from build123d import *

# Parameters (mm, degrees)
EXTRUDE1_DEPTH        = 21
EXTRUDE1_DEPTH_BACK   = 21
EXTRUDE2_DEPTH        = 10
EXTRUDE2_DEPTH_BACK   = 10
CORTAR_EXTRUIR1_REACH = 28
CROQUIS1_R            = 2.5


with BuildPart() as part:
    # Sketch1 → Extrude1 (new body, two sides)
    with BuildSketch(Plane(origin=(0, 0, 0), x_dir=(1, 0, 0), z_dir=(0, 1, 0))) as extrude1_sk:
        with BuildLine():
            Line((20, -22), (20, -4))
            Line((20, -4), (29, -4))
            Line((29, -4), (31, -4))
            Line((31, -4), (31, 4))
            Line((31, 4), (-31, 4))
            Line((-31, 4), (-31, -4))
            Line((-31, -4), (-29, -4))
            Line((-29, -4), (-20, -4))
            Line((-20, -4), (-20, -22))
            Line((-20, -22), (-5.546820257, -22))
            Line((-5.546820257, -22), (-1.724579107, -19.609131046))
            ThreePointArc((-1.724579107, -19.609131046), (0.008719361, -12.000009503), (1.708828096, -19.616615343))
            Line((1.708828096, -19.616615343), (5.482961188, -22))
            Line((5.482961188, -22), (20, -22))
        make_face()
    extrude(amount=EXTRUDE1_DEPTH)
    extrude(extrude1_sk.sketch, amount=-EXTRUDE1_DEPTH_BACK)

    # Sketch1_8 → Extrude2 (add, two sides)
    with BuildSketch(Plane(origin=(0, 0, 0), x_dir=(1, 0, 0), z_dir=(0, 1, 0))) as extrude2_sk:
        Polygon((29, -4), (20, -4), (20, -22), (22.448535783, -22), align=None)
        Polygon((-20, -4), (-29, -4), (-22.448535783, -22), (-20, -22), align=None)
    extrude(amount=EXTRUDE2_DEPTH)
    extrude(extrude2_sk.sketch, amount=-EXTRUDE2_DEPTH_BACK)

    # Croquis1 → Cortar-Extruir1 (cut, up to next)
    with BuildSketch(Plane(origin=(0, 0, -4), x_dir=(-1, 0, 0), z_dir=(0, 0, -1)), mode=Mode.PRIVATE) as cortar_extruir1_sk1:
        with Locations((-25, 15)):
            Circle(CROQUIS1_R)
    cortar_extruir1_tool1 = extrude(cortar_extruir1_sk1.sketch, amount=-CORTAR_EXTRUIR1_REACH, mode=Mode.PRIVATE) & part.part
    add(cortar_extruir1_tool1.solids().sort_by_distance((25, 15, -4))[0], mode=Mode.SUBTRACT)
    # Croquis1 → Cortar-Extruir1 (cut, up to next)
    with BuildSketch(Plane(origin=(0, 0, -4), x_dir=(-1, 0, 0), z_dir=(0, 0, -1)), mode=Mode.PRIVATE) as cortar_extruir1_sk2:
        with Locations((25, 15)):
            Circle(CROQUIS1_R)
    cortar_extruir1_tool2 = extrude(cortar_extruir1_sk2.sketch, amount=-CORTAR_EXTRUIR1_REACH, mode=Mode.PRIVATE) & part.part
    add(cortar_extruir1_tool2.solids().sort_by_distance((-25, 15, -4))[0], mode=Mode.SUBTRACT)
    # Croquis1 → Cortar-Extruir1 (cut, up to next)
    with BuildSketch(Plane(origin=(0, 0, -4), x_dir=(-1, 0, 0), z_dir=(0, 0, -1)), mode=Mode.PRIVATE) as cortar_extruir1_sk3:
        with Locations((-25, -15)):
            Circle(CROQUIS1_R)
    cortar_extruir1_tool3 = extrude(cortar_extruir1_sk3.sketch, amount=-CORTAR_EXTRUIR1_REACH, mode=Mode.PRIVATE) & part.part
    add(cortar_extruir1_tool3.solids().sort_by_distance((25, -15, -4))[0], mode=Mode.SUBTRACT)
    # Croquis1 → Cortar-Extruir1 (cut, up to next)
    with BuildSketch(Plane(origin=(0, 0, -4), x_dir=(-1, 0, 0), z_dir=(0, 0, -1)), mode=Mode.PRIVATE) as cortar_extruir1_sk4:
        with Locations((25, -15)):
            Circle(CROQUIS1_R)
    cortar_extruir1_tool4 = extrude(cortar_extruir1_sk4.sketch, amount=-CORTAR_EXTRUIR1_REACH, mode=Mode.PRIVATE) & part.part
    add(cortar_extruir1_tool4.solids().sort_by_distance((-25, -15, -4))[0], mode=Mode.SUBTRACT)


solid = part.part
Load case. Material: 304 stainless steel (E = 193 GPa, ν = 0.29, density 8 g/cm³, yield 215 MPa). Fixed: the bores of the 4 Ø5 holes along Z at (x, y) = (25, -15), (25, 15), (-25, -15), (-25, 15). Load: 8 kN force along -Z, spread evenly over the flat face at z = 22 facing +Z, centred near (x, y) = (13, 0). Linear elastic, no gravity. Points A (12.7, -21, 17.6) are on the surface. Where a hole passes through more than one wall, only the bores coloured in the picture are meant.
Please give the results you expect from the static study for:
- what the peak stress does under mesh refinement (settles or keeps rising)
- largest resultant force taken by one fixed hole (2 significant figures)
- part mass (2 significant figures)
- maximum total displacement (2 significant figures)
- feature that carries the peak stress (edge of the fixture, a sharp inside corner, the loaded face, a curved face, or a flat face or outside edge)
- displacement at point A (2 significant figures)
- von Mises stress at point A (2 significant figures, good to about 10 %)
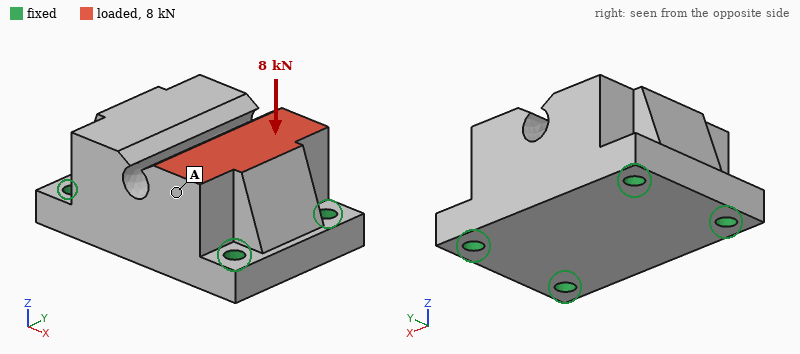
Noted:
keeps rising
3.3 kN
410 g
4.3 µm
edge of the fixture
3.9 µm
11 MPa
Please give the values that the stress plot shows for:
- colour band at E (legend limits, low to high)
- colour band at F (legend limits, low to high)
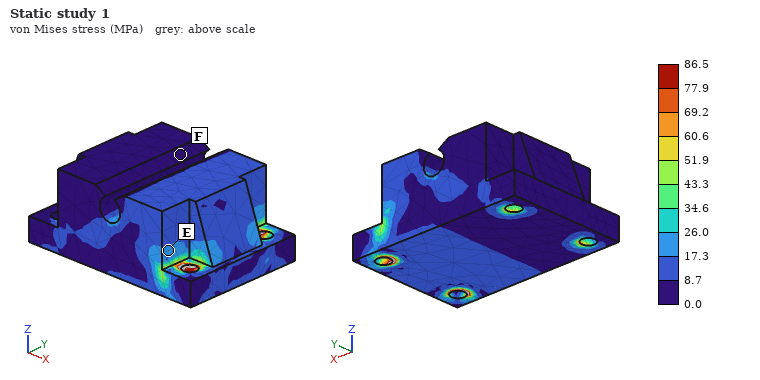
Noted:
17.3 to 26.0 MPa
0.0 to 8.7 MPa
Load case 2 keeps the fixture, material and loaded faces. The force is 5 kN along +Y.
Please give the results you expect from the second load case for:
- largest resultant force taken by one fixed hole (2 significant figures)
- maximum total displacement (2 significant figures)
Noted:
3.1 kN
8.3 µm
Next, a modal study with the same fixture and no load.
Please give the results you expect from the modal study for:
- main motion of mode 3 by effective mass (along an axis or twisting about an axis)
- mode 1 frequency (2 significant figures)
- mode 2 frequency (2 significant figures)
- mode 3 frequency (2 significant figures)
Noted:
along X
13 kHz
13 kHz
19 kHz
